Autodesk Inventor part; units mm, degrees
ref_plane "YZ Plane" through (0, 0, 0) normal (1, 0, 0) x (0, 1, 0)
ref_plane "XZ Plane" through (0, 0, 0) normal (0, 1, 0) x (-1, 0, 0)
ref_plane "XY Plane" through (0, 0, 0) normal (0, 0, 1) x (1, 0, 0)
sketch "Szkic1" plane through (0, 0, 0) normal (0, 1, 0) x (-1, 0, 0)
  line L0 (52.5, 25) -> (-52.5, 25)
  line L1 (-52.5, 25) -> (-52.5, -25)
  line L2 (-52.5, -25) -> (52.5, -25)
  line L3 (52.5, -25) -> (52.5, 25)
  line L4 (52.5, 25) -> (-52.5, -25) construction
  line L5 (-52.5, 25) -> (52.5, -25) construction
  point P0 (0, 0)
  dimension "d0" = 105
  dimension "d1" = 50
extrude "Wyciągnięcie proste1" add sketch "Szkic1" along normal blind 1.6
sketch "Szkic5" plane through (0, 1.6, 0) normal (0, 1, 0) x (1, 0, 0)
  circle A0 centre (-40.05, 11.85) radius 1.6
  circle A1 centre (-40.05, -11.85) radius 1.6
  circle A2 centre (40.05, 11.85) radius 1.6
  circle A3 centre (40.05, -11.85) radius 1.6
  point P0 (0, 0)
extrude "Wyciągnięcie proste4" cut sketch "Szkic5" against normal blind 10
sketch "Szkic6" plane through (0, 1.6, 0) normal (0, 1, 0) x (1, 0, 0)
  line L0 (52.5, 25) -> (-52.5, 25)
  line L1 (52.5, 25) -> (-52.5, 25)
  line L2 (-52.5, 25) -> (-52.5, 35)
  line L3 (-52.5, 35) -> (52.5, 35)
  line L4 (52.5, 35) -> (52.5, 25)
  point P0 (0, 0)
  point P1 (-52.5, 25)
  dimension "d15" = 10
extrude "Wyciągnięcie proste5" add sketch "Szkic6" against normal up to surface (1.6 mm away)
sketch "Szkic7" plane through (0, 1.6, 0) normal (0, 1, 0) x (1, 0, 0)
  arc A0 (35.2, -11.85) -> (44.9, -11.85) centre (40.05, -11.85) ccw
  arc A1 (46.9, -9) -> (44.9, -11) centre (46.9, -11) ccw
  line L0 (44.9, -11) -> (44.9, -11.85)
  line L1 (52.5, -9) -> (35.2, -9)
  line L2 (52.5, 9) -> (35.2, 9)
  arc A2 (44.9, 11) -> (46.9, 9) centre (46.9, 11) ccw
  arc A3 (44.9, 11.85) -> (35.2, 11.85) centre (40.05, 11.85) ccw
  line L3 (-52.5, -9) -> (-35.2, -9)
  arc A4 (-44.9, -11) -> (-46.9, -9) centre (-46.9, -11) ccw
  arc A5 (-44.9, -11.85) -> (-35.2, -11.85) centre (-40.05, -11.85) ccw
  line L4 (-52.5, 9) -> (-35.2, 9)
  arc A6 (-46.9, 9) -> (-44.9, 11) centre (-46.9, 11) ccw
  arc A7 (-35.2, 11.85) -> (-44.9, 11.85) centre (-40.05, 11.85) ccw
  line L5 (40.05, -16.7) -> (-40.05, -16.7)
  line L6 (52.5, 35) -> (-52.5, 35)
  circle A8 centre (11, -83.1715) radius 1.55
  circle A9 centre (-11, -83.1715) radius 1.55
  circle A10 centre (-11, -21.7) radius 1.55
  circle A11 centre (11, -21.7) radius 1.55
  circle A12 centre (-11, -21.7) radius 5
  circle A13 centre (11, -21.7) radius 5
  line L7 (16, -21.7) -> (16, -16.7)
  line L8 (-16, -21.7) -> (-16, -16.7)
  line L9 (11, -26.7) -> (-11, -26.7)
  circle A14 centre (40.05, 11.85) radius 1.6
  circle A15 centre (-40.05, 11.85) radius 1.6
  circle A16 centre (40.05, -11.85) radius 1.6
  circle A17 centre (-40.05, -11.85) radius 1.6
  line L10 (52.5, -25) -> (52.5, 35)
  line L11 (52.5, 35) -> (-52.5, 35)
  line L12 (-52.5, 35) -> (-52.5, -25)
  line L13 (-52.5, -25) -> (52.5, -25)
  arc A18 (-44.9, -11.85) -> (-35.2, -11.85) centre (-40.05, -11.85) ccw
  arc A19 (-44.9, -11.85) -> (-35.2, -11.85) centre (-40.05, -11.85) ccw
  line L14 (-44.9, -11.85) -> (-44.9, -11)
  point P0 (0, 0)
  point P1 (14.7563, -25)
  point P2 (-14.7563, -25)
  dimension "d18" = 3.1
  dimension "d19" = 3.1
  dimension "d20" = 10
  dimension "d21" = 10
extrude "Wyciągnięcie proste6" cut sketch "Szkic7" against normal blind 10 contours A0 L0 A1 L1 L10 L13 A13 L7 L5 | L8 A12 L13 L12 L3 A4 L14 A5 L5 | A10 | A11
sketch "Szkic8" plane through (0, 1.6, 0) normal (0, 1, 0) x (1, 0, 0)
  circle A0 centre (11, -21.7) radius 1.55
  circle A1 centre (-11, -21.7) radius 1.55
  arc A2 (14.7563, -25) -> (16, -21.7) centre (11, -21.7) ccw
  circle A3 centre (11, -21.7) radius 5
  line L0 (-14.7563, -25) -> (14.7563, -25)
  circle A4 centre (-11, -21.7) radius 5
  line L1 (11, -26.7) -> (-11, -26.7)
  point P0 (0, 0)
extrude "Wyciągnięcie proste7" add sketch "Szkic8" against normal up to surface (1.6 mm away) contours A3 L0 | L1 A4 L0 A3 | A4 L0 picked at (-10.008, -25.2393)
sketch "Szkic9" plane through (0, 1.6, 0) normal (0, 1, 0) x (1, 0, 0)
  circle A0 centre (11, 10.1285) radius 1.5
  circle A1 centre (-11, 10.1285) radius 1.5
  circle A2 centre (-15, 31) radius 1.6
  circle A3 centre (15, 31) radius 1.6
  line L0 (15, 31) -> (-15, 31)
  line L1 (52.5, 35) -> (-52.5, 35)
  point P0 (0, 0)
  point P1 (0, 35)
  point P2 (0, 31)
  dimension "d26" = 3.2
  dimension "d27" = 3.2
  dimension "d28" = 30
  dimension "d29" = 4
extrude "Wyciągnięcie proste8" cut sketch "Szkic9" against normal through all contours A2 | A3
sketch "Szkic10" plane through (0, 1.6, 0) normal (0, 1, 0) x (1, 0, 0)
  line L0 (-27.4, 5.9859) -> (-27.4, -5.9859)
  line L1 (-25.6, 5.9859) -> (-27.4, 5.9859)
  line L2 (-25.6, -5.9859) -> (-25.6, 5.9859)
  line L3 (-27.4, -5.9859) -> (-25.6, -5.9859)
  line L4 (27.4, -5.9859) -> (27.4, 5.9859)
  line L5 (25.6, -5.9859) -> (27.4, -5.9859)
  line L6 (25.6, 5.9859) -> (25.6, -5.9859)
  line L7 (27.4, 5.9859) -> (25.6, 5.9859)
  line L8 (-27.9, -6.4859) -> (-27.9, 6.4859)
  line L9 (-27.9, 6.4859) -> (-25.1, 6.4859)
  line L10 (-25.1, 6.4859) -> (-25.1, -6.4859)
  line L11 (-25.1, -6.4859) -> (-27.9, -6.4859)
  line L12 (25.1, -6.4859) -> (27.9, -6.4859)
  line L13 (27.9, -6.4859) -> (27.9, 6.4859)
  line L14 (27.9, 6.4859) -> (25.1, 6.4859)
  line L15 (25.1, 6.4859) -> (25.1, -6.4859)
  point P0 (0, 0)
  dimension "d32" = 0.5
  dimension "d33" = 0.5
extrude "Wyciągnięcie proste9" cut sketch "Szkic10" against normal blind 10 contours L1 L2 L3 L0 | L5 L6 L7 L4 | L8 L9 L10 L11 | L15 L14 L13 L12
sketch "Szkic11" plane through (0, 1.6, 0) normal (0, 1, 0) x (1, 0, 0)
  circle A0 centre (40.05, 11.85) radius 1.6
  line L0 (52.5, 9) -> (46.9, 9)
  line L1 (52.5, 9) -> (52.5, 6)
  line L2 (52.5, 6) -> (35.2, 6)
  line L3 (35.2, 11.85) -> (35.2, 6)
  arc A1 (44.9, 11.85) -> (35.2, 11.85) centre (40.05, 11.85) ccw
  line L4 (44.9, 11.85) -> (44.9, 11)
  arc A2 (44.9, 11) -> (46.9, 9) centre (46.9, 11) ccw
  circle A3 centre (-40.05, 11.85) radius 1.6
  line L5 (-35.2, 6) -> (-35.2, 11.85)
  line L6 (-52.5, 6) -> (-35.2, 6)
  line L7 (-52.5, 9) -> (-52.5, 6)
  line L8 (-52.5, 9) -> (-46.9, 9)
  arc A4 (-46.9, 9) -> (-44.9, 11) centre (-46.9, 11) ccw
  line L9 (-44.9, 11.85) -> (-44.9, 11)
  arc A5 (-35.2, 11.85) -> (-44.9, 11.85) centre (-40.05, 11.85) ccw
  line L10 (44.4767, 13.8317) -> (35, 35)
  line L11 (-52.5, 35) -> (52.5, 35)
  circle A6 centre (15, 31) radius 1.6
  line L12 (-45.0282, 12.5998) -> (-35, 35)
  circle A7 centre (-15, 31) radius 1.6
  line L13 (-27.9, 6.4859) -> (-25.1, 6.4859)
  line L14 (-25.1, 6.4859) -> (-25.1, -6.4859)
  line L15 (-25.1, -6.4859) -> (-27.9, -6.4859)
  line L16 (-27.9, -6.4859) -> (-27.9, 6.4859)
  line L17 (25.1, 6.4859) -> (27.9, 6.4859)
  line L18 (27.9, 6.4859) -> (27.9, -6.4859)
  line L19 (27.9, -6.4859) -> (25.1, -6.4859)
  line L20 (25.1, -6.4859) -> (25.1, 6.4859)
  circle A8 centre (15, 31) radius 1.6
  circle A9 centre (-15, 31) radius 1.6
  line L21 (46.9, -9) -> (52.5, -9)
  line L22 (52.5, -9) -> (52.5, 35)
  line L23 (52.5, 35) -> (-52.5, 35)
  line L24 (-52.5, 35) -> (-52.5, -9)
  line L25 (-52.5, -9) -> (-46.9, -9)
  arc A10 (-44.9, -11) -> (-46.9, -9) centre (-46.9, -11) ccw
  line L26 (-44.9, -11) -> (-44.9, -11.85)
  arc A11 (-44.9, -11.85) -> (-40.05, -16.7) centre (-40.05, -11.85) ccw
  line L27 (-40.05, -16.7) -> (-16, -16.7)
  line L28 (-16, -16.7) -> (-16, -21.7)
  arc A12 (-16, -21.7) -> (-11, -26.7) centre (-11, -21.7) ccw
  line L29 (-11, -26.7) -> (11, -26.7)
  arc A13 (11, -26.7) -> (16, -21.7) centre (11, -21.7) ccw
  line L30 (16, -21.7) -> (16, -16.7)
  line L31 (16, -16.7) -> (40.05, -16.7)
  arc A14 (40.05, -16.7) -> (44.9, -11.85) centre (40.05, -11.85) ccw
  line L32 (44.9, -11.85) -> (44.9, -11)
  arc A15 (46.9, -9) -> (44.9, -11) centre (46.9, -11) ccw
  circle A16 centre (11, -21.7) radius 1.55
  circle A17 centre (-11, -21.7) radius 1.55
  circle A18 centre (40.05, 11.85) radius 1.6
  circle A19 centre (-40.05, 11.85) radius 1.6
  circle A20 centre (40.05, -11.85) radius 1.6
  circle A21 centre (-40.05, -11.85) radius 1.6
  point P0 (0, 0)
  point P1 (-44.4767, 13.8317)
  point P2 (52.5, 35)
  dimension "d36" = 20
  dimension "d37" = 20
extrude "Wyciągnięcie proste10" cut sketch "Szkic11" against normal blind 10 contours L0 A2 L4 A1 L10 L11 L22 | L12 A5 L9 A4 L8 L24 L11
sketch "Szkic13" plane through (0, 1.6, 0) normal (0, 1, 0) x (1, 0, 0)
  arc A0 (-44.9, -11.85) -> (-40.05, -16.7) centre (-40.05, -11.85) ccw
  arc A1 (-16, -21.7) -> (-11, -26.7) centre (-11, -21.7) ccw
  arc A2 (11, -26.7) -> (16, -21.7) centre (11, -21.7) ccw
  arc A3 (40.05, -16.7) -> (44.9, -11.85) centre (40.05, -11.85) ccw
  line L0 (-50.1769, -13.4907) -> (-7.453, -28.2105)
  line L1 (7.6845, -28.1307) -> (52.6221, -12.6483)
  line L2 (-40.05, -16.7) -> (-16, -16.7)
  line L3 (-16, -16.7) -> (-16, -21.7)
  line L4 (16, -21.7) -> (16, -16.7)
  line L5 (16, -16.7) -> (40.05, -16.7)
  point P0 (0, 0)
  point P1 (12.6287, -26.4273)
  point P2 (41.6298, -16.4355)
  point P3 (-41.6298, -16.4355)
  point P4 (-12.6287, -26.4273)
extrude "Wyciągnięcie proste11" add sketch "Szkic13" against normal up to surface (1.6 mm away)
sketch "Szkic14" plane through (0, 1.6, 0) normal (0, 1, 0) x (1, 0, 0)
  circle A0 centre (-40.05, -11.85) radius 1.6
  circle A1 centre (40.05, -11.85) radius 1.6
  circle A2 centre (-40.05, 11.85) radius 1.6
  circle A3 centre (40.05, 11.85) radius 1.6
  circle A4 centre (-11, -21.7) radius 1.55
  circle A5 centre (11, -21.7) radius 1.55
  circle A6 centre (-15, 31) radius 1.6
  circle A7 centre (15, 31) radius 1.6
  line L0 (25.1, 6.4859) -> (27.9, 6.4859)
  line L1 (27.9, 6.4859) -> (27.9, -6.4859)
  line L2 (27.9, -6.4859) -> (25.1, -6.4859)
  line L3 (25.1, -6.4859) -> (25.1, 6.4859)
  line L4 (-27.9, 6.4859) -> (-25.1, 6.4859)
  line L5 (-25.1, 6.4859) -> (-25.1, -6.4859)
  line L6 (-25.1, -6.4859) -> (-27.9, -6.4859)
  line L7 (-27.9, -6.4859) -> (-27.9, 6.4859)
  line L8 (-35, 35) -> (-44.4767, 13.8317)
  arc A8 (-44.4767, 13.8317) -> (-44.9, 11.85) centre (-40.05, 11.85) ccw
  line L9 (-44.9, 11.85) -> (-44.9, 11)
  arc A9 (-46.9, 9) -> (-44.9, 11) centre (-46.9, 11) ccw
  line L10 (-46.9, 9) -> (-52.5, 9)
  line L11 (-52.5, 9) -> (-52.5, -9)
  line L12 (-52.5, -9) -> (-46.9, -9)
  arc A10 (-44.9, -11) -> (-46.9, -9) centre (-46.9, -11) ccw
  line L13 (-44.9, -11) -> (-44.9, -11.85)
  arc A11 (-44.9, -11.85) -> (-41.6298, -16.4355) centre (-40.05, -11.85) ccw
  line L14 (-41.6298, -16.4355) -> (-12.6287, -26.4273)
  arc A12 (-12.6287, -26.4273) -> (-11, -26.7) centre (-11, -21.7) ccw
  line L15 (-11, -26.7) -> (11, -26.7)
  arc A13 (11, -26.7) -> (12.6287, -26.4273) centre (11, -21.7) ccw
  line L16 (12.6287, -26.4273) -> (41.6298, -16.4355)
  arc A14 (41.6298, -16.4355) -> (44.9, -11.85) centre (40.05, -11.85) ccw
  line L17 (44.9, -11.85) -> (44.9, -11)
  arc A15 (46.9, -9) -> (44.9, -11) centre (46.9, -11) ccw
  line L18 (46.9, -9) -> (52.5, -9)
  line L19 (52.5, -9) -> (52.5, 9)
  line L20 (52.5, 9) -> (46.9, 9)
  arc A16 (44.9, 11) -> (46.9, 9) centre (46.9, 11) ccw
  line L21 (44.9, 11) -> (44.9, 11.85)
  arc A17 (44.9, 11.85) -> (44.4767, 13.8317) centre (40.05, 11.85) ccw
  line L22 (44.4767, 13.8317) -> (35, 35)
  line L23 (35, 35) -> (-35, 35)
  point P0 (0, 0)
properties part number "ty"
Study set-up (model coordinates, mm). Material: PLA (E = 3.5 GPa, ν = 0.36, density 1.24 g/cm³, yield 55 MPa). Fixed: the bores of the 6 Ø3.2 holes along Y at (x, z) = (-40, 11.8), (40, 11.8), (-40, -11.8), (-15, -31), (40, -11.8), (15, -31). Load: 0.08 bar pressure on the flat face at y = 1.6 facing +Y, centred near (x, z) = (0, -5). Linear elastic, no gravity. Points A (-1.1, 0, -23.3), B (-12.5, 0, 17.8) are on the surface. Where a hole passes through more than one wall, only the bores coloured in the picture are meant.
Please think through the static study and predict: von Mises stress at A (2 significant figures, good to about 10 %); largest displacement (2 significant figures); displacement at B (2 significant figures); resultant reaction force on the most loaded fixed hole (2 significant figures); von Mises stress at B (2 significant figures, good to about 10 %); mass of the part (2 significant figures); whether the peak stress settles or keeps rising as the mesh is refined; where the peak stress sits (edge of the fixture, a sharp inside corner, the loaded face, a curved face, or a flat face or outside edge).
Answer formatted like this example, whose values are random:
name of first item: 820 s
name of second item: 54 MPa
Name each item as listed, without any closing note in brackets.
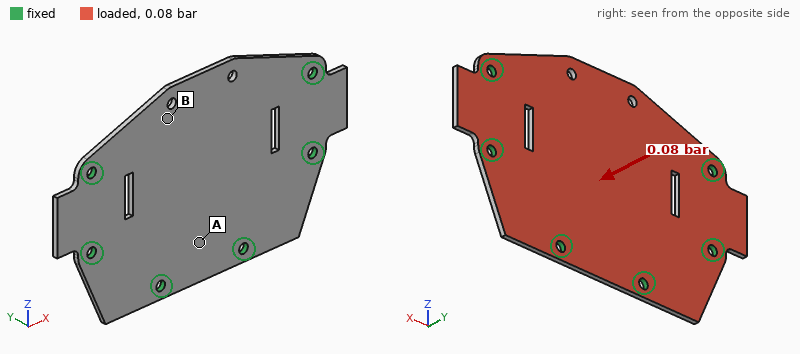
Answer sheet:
von Mises stress at A: 2.1 MPa
largest displacement: 0.94 mm
displacement at B: 0.64 mm
resultant reaction force on the most loaded fixed hole: 8.9 N
von Mises stress at B: 4.1 MPa
mass of the part: 10 g
whether the peak stress settles or keeps rising as the mesh is refined: keeps rising
where the peak stress sits: edge of the fixture
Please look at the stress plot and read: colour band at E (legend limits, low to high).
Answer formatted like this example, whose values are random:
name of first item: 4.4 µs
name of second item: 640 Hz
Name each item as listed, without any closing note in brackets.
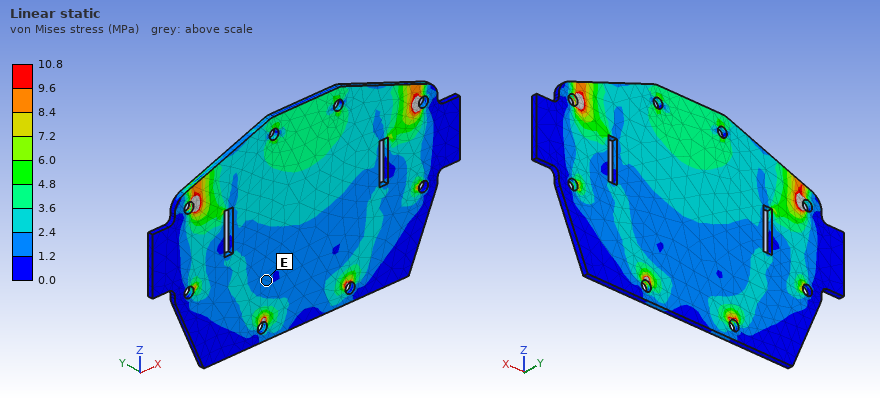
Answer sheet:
colour band at E: 1.2 to 2.4 MPa
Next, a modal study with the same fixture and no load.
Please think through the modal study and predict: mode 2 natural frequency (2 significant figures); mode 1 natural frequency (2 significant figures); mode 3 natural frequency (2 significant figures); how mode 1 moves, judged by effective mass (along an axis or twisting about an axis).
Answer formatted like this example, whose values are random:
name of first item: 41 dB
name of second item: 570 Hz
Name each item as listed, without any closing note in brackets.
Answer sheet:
mode 2 natural frequency: 1100 Hz
mode 1 natural frequency: 440 Hz
mode 3 natural frequency: 1200 Hz
how mode 1 moves, judged by effective mass: along Y
